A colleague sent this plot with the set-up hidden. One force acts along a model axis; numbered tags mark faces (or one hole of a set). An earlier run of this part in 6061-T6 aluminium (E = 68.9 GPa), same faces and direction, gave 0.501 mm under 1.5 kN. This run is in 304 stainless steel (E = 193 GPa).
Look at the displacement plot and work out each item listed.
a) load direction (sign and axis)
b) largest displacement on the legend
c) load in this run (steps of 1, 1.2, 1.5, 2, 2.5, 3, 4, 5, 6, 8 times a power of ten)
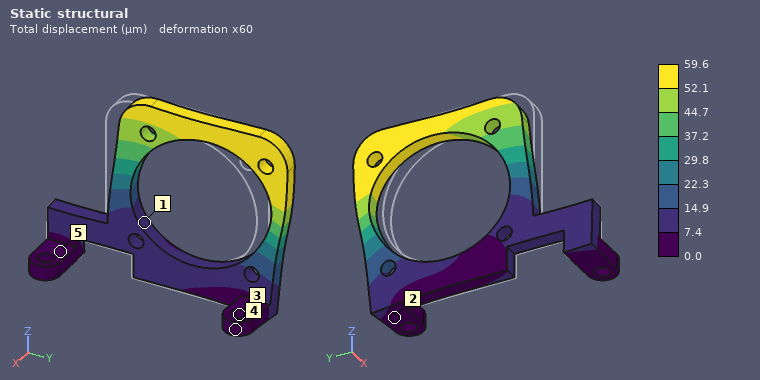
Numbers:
+Y
59.6 µm
500 N
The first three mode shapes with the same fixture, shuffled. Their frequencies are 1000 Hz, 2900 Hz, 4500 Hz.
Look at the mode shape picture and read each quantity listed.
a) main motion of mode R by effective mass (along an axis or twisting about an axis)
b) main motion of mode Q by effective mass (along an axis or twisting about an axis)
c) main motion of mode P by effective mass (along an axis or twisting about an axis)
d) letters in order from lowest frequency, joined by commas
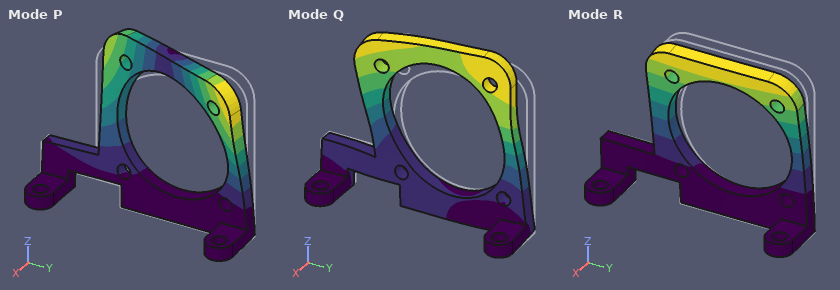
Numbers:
along X
along Y
twisting about Z
R, P, Q
